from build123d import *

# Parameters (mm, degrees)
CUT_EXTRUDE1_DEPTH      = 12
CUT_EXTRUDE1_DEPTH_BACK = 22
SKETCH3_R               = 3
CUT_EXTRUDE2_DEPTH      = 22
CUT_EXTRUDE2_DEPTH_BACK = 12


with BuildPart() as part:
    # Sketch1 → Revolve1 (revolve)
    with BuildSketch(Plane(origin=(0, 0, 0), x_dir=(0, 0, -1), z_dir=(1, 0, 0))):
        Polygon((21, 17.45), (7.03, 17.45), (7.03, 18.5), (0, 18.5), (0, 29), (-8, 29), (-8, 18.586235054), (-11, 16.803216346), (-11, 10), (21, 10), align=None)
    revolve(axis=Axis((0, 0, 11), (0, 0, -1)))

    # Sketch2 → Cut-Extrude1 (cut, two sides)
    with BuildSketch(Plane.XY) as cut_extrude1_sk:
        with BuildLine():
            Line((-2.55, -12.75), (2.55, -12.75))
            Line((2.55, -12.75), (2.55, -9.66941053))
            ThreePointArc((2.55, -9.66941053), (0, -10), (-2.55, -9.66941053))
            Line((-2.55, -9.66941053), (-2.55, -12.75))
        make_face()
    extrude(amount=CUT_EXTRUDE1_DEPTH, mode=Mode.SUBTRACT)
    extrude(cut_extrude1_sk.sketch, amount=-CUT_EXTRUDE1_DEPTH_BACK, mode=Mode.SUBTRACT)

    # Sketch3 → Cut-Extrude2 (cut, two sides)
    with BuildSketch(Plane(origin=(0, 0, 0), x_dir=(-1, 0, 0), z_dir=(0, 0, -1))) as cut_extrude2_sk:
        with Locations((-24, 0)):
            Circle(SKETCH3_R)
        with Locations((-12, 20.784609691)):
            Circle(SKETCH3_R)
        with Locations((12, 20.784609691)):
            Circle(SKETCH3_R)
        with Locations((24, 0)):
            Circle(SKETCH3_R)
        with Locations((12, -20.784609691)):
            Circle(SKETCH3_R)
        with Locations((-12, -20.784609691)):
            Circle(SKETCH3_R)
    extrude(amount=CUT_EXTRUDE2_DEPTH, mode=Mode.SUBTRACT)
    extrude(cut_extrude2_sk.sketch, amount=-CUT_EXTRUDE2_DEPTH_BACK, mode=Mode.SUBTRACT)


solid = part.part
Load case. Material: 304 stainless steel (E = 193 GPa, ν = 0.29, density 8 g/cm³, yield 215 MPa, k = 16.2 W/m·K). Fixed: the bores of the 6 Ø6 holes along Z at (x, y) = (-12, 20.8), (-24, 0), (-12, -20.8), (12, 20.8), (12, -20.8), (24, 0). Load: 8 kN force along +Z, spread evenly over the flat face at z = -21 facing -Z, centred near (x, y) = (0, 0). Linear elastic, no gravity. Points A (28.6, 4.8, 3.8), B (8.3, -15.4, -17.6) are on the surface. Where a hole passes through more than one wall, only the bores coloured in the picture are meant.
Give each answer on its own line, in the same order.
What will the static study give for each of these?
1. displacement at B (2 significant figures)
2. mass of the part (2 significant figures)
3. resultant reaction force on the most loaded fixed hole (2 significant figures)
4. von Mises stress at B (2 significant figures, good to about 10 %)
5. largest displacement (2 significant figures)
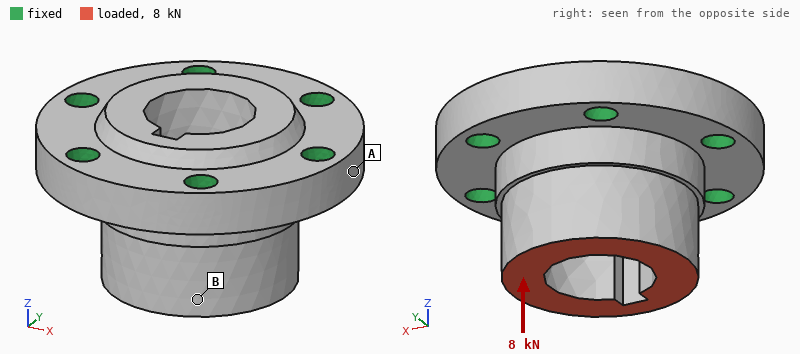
2.5 µm
270 g
1.4 kN
12 MPa
2.8 µm
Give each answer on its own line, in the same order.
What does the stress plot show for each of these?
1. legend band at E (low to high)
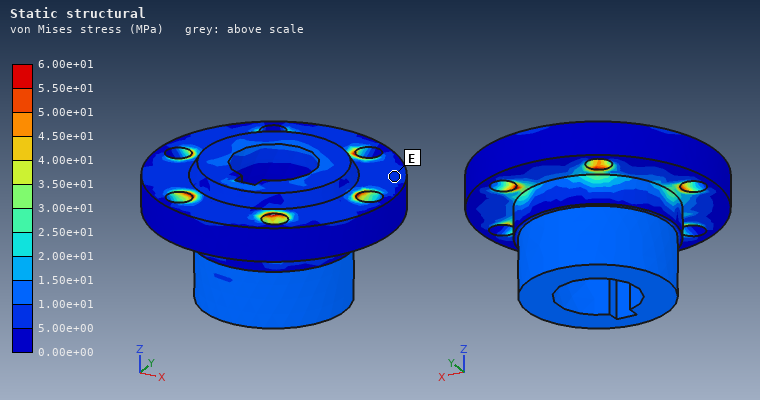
5.00e+00 to 1.00e+01 MPa
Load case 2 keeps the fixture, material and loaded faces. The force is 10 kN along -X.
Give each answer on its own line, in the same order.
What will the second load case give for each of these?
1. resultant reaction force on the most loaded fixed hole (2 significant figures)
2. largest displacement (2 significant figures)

4.5 kN
19 µm
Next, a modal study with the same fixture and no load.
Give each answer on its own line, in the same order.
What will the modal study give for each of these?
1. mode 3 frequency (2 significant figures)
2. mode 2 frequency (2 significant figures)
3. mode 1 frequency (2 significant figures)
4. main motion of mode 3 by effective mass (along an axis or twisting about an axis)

26 kHz
20 kHz
20 kHz
along Z
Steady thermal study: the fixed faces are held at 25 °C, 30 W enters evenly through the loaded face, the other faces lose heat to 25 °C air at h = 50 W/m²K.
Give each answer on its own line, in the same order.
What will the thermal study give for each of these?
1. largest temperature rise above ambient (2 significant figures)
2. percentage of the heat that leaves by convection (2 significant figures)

66 K
29 %
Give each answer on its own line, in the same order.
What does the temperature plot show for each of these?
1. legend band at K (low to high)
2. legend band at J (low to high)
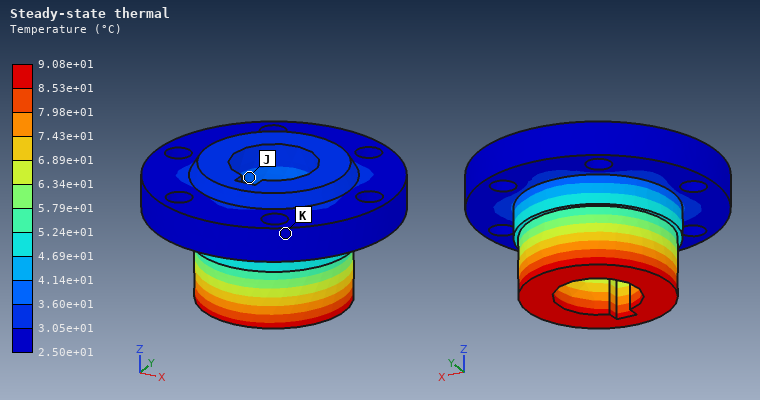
2.50e+01 to 3.05e+01 °C
3.60e+01 to 4.14e+01 °C
